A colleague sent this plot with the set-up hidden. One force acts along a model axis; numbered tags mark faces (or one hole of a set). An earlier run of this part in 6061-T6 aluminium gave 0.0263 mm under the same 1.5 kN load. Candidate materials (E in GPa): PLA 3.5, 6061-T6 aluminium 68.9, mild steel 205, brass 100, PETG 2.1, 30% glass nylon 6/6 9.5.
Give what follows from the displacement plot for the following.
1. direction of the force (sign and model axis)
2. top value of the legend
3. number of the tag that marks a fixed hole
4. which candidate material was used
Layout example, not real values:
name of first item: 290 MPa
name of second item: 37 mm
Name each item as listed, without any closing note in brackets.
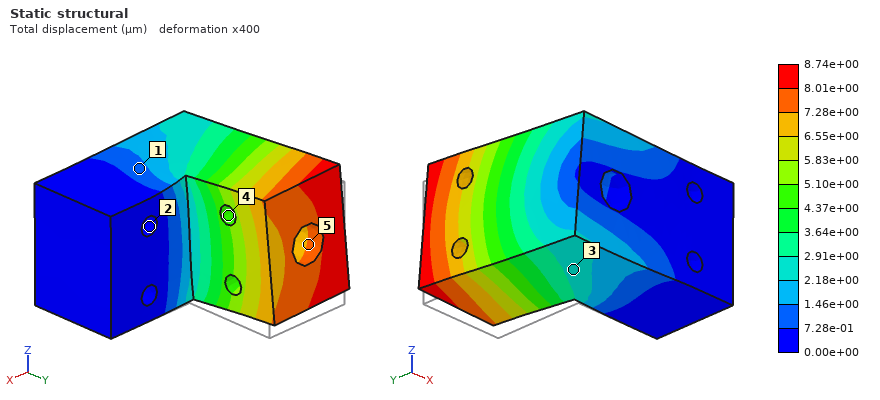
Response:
direction of the force: +Z
top value of the legend: 8.74e+00 µm
number of the tag that marks a fixed hole: 2
which candidate material was used: mild steel
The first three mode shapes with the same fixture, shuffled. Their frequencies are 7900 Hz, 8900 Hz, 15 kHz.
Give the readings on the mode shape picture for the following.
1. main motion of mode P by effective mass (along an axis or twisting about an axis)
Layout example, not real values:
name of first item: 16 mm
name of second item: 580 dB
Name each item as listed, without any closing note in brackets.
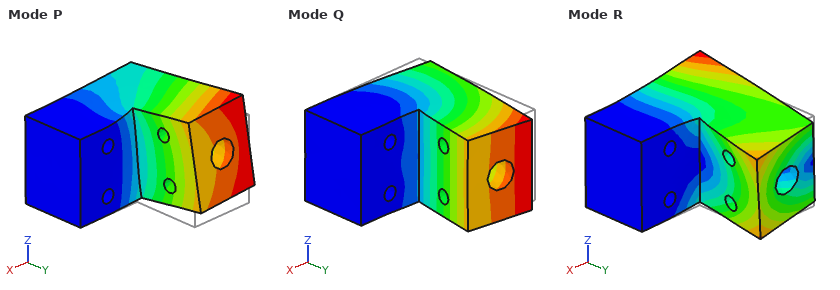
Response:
main motion of mode P by effective mass: along Z
